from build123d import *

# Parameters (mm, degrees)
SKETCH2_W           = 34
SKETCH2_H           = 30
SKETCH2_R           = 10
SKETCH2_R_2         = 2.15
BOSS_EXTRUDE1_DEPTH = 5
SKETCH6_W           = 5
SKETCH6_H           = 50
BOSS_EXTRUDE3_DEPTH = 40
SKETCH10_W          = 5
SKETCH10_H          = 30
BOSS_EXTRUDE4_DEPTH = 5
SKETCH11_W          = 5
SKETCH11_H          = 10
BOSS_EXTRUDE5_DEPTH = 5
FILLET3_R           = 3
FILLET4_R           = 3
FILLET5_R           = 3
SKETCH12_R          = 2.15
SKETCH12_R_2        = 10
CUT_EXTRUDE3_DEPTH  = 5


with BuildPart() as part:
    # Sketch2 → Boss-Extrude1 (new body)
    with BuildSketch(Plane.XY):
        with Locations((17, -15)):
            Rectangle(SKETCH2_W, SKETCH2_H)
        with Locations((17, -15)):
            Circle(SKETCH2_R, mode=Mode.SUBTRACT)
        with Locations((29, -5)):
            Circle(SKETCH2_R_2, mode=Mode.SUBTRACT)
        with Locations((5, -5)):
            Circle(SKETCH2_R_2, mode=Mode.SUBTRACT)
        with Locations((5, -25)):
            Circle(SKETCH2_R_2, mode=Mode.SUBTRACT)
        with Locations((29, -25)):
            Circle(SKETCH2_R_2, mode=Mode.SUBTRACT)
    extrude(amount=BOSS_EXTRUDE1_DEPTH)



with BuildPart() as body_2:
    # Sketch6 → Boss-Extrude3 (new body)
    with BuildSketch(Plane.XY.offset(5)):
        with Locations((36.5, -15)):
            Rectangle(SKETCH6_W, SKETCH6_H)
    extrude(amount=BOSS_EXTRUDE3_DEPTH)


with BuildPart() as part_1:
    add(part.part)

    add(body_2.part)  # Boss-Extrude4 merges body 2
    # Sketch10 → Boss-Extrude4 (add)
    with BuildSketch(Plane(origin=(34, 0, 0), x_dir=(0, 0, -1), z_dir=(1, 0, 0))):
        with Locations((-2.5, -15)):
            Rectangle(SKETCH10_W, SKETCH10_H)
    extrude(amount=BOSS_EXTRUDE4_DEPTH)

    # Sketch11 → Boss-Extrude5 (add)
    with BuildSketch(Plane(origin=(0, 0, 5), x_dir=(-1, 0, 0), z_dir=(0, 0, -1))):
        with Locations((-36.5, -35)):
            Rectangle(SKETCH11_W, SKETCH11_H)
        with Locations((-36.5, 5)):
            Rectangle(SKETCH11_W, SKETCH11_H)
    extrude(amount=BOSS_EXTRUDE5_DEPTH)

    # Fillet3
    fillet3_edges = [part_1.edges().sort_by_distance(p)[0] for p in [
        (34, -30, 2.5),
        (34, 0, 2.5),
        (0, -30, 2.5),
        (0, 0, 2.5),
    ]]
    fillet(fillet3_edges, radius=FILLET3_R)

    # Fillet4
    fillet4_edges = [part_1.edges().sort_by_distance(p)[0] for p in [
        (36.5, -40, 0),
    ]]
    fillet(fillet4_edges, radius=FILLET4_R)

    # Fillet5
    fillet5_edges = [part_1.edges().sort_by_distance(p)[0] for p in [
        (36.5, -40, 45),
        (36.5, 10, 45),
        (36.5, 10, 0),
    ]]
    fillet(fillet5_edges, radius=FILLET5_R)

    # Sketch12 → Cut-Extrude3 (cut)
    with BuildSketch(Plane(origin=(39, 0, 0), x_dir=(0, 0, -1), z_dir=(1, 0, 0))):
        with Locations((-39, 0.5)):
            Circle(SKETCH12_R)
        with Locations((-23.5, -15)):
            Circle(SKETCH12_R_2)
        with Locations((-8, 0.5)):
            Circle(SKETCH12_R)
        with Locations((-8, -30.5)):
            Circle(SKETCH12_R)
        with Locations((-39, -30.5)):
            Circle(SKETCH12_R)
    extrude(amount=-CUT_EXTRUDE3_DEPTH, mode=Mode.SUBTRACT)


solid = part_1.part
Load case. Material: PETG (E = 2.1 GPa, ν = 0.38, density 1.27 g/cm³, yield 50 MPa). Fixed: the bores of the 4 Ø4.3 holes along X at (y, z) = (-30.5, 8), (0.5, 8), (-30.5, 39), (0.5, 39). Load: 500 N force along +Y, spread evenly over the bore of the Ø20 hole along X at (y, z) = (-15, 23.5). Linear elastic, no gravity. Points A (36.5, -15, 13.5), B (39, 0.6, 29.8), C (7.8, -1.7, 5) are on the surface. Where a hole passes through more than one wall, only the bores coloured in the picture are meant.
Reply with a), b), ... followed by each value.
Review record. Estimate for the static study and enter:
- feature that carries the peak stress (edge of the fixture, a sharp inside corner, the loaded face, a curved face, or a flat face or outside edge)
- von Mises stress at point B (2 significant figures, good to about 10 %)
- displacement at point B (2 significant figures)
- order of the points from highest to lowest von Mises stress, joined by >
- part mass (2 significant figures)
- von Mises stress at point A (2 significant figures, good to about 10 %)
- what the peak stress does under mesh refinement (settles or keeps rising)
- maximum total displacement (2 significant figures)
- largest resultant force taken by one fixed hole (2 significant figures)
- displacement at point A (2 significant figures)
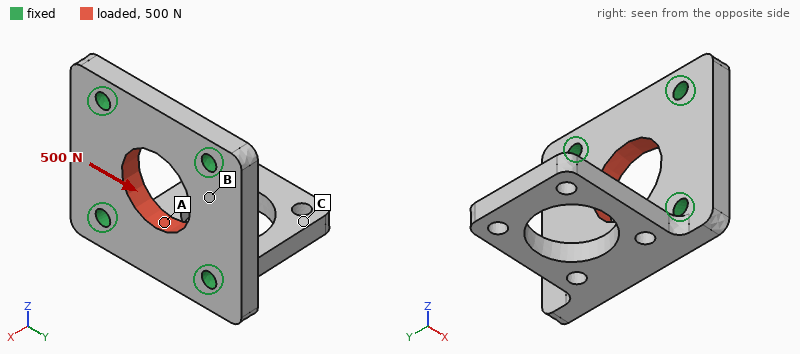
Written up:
a) edge of the fixture
b) 1.4 MPa
c) 14 µm
d) A > B > C
e) 16 g
f) 2.7 MPa
g) keeps rising
h) 22 µm
i) 130 N
j) 13 µm
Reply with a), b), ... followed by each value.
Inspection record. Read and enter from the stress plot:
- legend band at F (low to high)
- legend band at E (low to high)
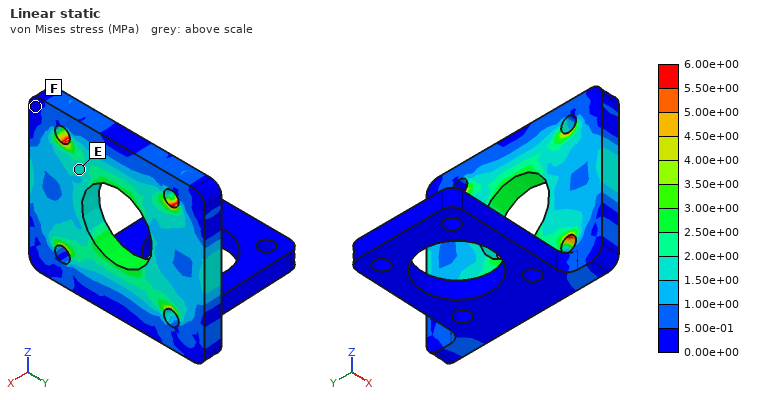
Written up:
a) 0.00e+00 to 5.00e-01 MPa
b) 1.50e+00 to 2.00e+00 MPa
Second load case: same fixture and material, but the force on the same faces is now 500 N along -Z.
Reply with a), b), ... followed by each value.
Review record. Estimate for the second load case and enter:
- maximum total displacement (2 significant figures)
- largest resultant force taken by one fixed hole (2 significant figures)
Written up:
a) 26 µm
b) 130 N
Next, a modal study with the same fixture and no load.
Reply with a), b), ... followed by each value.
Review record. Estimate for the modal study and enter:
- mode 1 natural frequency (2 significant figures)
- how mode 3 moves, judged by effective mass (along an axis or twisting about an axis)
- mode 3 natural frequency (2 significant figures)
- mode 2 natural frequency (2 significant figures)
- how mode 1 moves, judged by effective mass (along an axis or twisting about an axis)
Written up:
a) 620 Hz
b) along Y
c) 2100 Hz
d) 1600 Hz
e) along Z
